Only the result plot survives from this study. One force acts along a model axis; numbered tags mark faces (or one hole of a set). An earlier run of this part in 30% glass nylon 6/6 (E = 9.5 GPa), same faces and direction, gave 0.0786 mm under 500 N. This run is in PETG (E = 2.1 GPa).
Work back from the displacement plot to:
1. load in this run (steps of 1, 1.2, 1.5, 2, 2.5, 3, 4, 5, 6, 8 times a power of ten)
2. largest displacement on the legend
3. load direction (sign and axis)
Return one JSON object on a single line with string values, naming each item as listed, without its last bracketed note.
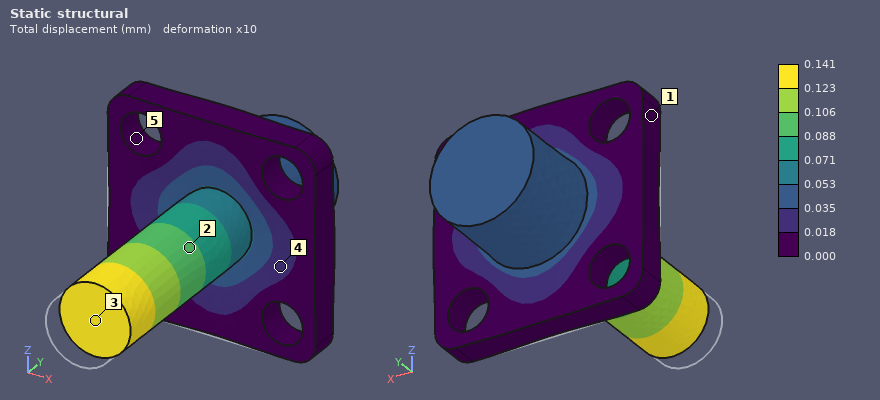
{"load in this run": "200 N", "largest displacement on the legend": "0.141 mm", "load direction": "+Y"}
